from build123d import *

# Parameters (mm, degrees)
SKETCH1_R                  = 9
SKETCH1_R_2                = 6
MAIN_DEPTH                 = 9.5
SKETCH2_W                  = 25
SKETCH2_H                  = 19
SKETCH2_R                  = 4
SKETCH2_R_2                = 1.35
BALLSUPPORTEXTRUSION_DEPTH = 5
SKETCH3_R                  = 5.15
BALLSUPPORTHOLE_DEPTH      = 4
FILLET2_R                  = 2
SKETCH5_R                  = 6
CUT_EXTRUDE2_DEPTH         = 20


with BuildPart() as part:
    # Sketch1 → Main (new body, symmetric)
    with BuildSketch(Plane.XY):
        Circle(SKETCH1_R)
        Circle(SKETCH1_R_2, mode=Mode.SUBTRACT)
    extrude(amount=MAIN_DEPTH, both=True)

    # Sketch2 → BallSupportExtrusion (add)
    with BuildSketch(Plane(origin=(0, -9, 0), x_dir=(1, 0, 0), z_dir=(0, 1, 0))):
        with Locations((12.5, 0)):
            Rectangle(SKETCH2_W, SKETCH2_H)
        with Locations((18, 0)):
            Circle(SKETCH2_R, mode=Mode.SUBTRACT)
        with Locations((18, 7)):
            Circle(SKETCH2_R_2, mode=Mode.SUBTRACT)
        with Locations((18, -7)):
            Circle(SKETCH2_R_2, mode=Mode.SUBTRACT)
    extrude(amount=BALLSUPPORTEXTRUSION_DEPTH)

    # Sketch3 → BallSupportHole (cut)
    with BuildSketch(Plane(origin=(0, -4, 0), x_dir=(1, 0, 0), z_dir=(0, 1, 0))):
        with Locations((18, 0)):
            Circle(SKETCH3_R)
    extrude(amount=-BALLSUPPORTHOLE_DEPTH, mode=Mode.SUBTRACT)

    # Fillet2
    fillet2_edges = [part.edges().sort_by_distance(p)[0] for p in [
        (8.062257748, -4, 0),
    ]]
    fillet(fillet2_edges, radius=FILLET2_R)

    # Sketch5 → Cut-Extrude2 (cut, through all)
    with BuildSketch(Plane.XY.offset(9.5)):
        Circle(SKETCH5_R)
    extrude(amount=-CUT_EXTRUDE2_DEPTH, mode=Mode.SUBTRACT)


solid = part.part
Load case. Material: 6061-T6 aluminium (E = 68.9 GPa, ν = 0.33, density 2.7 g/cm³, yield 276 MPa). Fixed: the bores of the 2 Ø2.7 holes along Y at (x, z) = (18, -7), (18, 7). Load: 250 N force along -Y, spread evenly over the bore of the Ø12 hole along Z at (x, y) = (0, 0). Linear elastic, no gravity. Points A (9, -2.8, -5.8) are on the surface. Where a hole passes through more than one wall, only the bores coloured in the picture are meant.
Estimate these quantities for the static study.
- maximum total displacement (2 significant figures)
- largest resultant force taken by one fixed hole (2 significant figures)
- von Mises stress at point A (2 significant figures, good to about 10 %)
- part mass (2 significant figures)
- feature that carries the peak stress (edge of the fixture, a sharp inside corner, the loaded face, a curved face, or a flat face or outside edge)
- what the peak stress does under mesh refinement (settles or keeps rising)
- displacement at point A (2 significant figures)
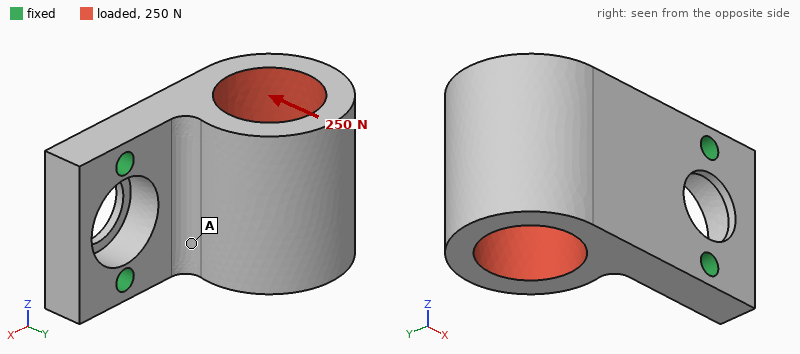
90 µm
130 N
14 MPa
11 g
edge of the fixture
keeps rising
21 µm
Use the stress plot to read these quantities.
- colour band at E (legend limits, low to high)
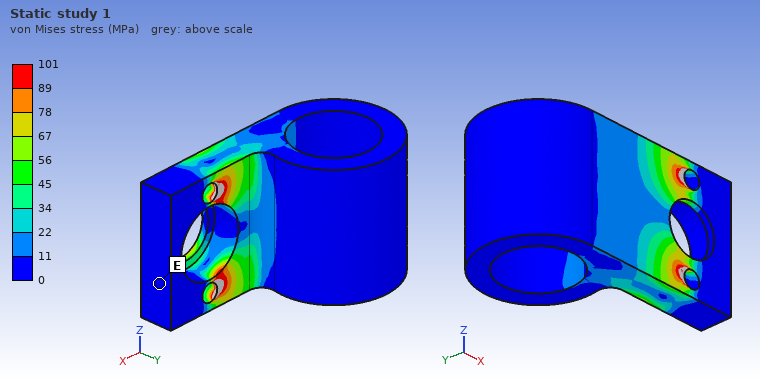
0 to 11 MPa
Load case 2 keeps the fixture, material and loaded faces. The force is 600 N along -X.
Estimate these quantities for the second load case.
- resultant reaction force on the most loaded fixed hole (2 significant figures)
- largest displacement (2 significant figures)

310 N
0.11 mm
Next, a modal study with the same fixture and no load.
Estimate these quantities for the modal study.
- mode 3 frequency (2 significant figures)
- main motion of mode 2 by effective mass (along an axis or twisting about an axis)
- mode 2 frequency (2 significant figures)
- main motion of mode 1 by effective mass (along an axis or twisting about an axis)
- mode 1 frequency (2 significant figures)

16 kHz
along Z
8600 Hz
along Y
3300 Hz
